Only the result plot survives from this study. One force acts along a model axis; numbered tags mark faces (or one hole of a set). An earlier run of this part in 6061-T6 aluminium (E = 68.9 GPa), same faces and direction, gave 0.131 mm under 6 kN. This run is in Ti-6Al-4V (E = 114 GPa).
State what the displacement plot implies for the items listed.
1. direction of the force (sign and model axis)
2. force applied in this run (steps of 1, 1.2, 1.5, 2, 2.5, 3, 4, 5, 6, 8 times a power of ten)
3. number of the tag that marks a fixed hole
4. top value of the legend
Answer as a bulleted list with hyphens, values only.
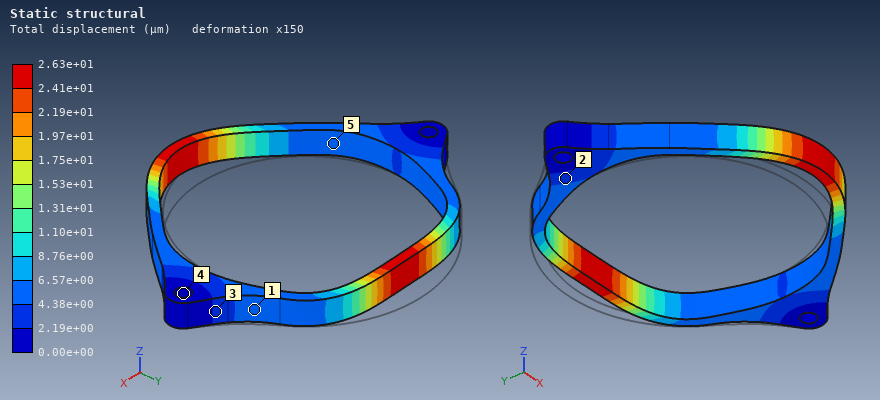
- -Y
- 2 kN
- 4
- 2.63e+01 µm
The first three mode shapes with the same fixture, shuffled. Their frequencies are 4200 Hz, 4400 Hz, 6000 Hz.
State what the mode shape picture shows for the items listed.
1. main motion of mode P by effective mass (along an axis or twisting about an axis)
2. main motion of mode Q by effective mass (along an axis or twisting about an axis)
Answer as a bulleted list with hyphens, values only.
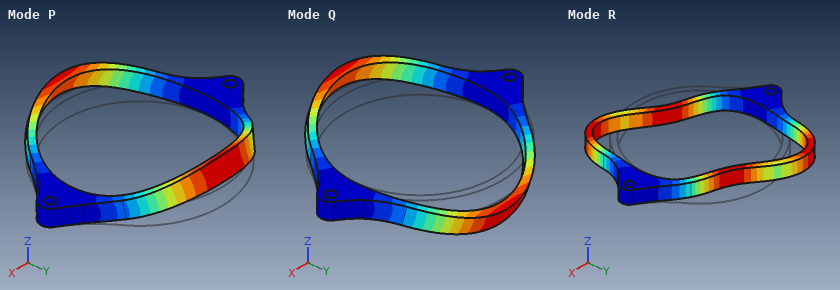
- along Z
- twisting about X
